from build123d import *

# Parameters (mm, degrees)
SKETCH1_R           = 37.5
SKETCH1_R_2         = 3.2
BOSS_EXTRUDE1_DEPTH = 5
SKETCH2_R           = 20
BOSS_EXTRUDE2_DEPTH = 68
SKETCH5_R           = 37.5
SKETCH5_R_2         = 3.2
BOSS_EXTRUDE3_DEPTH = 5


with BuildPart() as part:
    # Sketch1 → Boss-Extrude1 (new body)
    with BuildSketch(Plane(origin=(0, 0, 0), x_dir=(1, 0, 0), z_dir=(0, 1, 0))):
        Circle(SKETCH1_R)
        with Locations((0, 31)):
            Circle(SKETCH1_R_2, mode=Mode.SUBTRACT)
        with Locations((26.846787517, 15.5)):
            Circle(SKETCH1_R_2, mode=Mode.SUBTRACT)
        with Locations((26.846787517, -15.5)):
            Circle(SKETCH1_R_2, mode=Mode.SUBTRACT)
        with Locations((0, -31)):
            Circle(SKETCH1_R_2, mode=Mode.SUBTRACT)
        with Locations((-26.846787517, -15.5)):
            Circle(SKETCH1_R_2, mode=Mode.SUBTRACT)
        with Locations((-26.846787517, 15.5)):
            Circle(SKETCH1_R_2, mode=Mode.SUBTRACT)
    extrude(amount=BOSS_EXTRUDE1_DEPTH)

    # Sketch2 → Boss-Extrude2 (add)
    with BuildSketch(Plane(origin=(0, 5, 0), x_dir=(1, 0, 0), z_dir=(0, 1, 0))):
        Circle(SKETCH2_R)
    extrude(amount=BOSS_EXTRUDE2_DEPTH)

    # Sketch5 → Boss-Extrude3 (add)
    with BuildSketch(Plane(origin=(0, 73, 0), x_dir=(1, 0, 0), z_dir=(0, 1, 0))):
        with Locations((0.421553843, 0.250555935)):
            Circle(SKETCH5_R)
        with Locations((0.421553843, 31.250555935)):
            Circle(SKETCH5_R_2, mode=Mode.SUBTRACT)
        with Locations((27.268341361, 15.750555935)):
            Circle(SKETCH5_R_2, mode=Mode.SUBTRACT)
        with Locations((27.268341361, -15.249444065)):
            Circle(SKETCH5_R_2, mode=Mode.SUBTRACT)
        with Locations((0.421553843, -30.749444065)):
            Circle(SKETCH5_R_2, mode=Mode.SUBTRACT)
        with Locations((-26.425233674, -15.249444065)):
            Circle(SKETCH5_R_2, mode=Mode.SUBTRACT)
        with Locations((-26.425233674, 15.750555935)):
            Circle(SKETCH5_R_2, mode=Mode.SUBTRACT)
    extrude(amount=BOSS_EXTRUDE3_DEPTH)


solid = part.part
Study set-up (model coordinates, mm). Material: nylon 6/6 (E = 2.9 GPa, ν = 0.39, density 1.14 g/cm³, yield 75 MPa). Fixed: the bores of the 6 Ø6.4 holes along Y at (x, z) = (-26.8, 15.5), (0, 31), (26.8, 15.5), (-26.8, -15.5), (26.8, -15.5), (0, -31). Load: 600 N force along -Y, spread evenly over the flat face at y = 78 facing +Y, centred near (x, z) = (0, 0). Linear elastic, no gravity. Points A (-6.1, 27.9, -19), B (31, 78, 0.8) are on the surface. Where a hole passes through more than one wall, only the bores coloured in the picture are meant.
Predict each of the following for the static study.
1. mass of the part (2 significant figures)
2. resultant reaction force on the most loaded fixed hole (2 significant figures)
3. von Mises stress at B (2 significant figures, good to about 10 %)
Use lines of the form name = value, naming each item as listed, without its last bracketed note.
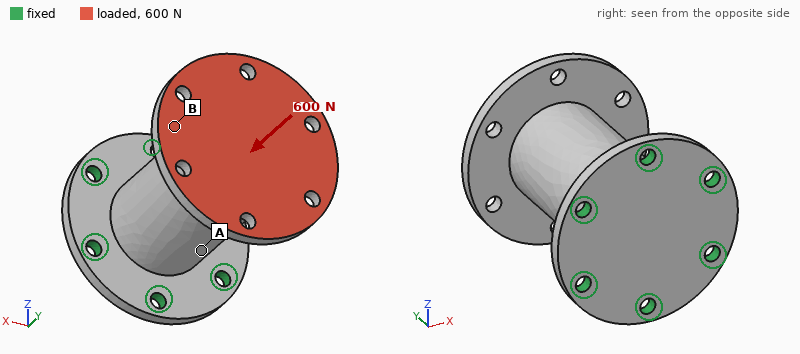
mass of the part = 150 g
resultant reaction force on the most loaded fixed hole = 110 N
von Mises stress at B = 1.3 MPa
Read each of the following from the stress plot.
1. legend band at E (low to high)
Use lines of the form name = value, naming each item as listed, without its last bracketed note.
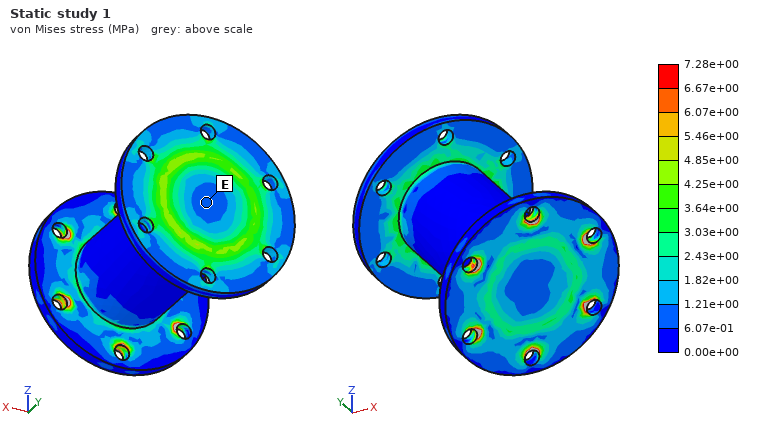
legend band at E = 6.07e-01 to 1.21e+00 MPa
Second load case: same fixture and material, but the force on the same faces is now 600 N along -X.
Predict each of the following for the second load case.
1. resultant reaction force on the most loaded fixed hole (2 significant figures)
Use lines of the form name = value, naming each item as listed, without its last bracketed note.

resultant reaction force on the most loaded fixed hole = 530 N
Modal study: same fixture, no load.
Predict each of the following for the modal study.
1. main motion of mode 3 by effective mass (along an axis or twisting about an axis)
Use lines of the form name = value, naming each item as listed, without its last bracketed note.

main motion of mode 3 by effective mass = along Y
